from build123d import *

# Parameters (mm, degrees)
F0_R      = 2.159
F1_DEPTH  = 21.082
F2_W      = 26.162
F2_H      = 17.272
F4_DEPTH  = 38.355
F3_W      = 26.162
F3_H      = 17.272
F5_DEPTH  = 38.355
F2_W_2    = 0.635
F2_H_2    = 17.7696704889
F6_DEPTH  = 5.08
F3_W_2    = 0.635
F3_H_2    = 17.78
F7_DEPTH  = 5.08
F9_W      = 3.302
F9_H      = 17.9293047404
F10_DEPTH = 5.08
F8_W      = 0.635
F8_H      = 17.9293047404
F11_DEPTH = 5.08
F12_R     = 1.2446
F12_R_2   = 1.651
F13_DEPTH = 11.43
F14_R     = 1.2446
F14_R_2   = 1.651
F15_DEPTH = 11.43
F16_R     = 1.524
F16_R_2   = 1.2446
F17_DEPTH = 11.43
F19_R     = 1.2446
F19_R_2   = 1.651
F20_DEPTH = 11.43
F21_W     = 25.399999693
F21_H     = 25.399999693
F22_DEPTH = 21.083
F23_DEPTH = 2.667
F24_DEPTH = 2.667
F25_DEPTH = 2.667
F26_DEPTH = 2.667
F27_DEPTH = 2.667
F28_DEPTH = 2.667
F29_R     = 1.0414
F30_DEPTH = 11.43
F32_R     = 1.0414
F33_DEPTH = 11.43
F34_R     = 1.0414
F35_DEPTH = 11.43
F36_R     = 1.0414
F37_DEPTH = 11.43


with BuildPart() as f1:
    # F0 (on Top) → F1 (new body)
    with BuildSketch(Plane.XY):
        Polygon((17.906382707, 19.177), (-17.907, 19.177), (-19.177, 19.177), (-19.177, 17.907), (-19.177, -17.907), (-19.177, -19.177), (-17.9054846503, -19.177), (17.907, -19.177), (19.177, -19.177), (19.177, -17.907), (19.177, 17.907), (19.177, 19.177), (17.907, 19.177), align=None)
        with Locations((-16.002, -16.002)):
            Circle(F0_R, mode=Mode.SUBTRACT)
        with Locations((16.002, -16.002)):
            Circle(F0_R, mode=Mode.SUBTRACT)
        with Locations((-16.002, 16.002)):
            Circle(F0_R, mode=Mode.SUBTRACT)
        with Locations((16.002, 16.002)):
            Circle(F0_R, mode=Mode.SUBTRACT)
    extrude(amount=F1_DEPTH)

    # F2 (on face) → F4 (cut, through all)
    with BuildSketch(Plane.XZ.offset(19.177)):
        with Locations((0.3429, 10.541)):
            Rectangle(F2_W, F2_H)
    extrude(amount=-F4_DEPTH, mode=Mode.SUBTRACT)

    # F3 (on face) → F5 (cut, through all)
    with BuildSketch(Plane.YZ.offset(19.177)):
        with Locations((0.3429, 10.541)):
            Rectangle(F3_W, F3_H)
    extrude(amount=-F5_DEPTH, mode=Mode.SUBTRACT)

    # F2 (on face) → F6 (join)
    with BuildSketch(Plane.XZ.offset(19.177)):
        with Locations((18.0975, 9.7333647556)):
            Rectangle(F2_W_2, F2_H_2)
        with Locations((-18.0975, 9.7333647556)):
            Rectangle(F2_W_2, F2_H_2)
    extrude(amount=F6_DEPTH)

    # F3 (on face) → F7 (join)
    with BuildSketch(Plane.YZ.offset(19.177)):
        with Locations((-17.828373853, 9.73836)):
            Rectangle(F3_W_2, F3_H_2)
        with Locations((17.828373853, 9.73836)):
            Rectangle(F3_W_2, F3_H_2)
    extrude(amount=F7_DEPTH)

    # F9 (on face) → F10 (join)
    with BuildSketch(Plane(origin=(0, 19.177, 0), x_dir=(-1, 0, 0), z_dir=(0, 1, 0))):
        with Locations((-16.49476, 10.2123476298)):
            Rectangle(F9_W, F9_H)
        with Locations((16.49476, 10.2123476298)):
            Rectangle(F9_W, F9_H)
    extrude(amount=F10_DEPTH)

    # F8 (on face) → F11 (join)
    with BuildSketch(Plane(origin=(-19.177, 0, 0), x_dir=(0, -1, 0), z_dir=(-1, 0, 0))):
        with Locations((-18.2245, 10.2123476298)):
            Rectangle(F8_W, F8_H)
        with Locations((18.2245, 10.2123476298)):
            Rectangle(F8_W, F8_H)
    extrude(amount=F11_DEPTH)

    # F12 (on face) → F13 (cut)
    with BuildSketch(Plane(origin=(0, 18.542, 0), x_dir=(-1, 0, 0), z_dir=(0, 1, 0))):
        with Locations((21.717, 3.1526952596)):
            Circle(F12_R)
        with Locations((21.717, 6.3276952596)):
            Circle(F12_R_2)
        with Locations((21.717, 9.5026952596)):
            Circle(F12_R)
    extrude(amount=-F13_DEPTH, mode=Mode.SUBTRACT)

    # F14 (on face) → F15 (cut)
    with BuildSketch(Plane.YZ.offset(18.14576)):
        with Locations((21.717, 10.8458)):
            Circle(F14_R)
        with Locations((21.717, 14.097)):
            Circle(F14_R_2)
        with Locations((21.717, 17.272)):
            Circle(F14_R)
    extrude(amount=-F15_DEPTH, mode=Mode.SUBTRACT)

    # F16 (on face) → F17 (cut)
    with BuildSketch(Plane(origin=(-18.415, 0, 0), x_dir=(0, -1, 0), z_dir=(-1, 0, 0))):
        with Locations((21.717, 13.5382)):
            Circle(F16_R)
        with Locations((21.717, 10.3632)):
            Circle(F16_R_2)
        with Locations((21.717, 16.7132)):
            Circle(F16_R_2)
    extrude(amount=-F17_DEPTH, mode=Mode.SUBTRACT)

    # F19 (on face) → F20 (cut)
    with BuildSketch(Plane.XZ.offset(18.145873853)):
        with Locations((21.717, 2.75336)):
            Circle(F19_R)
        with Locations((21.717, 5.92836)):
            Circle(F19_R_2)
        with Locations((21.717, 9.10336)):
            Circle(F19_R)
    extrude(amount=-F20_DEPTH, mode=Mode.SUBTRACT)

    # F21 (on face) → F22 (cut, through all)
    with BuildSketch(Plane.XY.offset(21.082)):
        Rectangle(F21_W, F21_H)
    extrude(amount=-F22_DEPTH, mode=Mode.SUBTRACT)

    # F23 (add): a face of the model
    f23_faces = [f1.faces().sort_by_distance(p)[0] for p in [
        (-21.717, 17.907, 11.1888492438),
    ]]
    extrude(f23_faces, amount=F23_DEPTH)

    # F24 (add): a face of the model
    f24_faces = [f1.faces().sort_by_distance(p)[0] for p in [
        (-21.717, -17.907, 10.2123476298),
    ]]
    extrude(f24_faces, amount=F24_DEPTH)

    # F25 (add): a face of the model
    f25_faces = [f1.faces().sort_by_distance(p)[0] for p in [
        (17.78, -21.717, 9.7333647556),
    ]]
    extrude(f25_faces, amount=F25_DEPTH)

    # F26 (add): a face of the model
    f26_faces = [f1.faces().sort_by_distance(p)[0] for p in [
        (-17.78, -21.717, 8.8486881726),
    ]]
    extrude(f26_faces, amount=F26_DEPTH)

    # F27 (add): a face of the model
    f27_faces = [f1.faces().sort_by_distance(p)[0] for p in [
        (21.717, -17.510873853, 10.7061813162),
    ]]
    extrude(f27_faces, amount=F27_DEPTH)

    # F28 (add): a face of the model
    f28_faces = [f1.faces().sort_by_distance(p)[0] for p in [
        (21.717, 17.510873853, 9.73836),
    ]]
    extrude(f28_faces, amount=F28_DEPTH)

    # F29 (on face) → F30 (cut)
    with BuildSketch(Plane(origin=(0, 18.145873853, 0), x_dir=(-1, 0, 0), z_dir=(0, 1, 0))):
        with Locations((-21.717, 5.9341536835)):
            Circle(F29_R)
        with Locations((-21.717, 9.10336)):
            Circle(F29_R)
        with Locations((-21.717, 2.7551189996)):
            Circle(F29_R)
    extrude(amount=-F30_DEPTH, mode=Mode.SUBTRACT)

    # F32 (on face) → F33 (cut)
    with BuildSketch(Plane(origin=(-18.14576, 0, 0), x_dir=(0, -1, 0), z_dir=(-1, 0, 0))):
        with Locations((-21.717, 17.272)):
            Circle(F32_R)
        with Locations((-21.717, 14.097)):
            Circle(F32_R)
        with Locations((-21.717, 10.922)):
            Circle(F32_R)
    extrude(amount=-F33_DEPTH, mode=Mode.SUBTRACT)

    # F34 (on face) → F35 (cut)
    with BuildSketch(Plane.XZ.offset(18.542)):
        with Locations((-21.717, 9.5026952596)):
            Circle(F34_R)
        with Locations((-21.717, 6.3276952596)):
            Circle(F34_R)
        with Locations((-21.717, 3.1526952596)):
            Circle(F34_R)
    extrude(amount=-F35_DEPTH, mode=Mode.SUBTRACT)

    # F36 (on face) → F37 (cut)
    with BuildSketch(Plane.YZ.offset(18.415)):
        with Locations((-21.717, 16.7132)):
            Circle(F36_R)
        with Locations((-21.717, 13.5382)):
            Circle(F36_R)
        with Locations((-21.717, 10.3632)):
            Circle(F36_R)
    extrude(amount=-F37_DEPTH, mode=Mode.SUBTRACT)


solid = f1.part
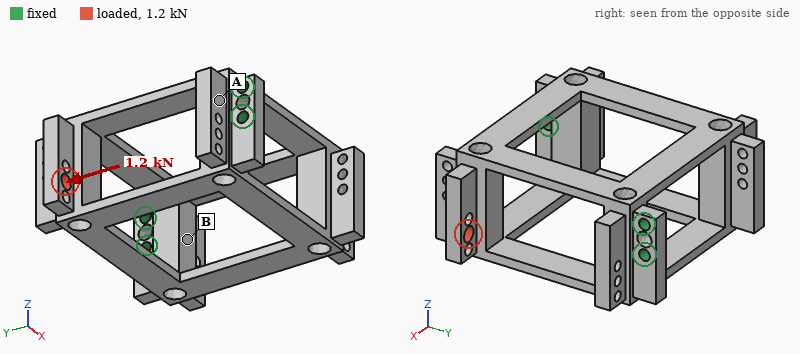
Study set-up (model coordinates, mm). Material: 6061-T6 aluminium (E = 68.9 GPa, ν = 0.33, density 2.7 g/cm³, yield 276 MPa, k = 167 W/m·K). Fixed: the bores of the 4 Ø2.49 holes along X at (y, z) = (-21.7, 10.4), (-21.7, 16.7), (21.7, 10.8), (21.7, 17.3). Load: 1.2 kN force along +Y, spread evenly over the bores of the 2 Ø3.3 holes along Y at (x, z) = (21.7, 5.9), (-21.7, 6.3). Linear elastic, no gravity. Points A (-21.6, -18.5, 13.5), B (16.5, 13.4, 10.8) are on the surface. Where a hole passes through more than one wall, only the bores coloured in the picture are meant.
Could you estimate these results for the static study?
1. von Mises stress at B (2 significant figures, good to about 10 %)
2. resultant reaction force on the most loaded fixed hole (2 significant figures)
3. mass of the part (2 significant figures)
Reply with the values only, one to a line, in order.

40 MPa
750 N
18 g
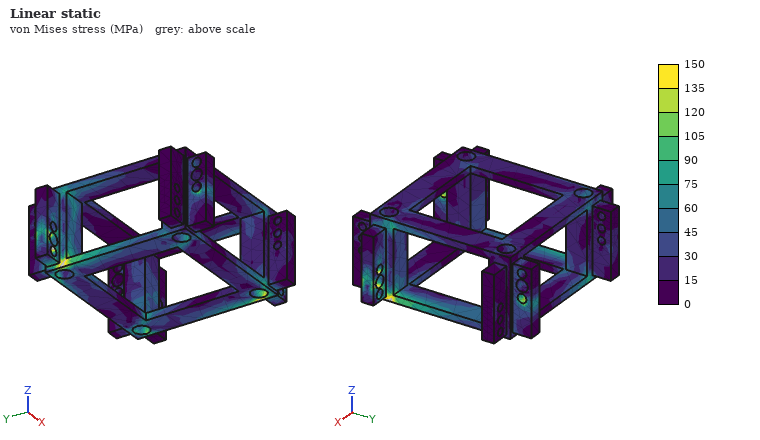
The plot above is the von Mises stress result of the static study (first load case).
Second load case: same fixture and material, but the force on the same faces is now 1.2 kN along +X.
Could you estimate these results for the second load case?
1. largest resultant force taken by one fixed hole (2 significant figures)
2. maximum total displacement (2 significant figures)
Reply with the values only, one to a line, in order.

710 N
87 µm
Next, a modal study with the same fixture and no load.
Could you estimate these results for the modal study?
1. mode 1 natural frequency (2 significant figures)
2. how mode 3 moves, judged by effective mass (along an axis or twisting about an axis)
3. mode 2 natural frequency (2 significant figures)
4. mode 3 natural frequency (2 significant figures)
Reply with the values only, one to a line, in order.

1700 Hz
along X
1700 Hz
8100 Hz
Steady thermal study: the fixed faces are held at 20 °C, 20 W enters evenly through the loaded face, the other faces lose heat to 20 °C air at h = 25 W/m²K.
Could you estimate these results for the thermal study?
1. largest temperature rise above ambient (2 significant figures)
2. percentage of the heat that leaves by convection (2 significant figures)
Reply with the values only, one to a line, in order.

59 K
25 %
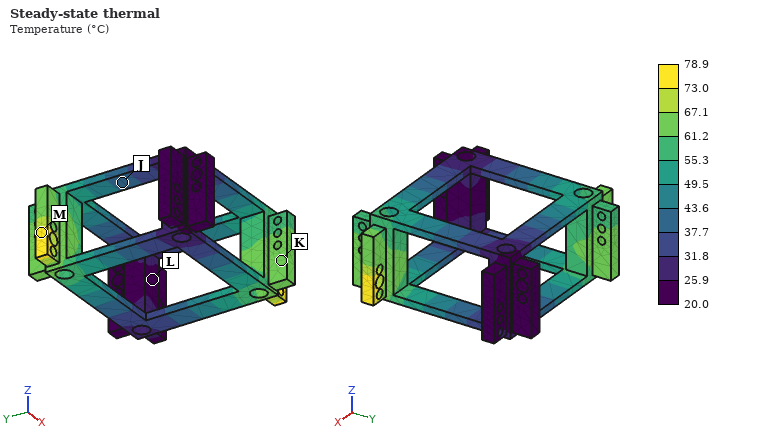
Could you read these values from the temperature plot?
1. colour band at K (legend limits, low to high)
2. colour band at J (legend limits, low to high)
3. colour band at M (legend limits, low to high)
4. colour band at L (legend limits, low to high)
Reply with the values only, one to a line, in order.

61.2 to 67.1 °C
37.7 to 43.6 °C
73.0 to 78.9 °C
20.0 to 25.9 °C
